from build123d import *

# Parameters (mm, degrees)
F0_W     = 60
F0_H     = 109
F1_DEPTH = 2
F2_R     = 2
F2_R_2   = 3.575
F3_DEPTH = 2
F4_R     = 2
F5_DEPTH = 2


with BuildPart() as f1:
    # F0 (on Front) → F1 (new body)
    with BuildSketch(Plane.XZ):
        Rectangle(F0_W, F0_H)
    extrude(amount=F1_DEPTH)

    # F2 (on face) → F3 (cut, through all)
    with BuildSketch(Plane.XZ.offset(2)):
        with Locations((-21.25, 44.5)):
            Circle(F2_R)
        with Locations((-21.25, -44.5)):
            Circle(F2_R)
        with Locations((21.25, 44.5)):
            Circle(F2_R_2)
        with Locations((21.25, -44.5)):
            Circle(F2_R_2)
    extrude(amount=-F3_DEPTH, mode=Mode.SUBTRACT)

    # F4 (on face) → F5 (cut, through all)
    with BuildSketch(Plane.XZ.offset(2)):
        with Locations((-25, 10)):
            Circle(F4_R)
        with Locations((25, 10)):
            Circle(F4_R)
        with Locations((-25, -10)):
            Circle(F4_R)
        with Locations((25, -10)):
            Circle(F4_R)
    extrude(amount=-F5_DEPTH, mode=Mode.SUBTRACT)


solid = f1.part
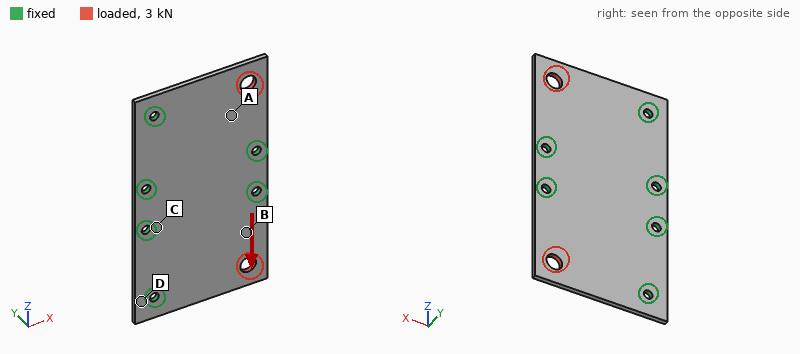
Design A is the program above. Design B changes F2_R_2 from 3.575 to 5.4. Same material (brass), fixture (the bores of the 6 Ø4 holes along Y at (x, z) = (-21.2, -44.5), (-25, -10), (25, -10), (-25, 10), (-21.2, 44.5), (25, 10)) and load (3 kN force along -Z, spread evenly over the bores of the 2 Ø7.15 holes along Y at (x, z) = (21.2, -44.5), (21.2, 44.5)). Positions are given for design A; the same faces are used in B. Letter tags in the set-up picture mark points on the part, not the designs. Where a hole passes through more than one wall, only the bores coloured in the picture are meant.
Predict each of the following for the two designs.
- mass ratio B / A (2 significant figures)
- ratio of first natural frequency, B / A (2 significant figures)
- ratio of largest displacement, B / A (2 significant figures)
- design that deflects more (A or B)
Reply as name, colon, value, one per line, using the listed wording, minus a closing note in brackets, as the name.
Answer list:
mass ratio B / A: 0.98
ratio of first natural frequency, B / A: 1.0
ratio of largest displacement, B / A: 1.3
design that deflects more: B
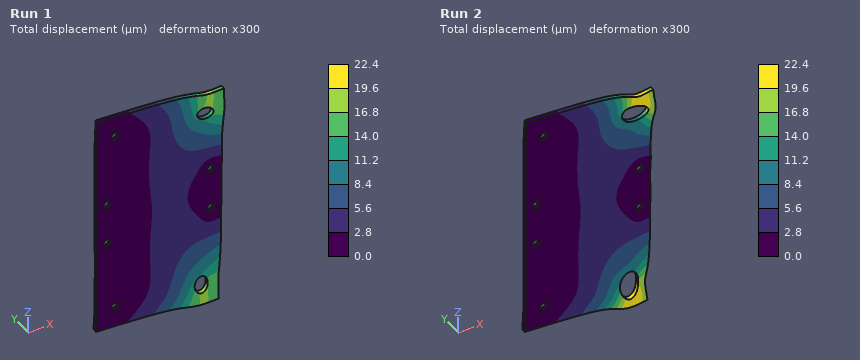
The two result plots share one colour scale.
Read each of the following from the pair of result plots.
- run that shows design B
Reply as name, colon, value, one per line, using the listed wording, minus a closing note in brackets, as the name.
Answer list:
run that shows design B: Run 2
